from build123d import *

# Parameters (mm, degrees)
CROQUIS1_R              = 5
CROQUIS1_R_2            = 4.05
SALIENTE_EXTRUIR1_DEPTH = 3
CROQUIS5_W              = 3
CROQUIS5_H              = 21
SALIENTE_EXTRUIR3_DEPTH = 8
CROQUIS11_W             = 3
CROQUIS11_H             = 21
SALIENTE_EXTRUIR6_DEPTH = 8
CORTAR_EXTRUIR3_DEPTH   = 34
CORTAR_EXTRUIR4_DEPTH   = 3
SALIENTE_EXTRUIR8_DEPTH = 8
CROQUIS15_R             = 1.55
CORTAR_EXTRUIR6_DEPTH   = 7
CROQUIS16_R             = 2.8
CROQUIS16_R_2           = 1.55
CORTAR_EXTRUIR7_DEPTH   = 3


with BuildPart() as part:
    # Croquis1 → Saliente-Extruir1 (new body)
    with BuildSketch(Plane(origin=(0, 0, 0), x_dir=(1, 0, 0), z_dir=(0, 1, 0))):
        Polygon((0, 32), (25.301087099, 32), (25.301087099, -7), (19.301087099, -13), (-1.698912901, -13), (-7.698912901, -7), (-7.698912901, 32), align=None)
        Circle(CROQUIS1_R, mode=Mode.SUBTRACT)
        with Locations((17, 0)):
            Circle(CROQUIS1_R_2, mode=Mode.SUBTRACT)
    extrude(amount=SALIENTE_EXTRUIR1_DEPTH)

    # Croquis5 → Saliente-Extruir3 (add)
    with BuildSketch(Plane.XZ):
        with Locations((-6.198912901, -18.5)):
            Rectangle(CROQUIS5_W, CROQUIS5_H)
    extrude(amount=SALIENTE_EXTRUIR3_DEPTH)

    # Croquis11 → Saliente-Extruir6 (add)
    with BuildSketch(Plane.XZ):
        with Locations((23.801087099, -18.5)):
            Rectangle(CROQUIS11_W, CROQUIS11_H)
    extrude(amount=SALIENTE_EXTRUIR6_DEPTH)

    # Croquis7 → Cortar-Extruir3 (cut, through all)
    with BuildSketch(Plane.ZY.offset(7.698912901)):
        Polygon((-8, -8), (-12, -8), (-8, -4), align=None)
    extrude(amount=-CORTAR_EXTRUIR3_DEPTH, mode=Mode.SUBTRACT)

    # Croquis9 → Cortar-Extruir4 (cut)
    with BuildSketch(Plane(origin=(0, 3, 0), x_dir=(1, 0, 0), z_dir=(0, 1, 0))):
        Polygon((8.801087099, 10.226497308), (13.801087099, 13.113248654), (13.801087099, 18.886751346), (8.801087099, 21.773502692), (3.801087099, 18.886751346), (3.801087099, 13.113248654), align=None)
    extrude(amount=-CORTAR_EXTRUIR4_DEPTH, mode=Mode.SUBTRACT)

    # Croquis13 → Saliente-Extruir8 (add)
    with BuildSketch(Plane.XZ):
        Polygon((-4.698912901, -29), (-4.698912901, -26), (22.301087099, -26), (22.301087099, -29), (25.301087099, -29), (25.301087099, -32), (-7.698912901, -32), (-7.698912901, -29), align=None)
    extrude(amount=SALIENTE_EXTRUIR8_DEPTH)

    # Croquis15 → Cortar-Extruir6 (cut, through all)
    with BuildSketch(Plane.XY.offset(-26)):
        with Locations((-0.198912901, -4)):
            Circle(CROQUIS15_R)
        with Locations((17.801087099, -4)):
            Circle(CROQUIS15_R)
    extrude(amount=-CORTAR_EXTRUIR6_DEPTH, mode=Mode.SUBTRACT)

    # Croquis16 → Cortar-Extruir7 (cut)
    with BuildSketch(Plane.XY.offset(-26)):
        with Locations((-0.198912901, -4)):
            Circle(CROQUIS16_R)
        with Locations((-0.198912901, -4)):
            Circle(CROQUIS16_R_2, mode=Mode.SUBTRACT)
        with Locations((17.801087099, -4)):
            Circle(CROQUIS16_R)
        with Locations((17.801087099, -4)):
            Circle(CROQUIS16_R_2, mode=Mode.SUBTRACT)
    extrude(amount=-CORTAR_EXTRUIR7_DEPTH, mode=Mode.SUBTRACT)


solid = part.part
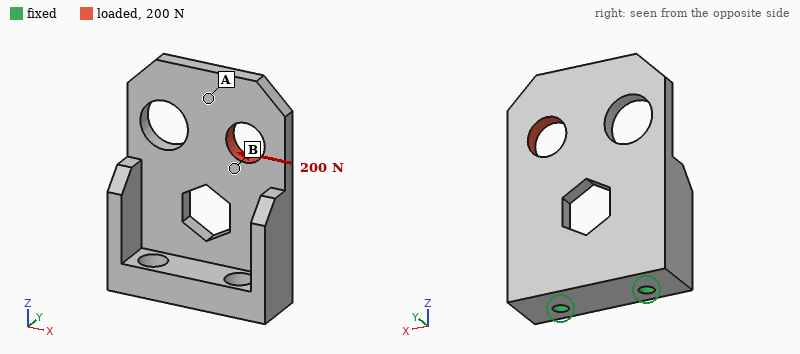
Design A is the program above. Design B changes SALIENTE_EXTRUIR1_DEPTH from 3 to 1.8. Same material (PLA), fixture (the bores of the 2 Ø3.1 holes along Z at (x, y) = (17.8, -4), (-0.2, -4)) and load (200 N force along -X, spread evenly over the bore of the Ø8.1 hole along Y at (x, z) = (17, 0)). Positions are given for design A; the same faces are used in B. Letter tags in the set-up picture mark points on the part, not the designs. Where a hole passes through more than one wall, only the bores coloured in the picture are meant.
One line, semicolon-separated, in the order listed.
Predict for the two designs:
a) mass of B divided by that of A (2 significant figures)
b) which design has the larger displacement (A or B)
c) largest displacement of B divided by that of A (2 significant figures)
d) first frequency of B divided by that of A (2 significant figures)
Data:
0.75; B; 1.3; 0.85
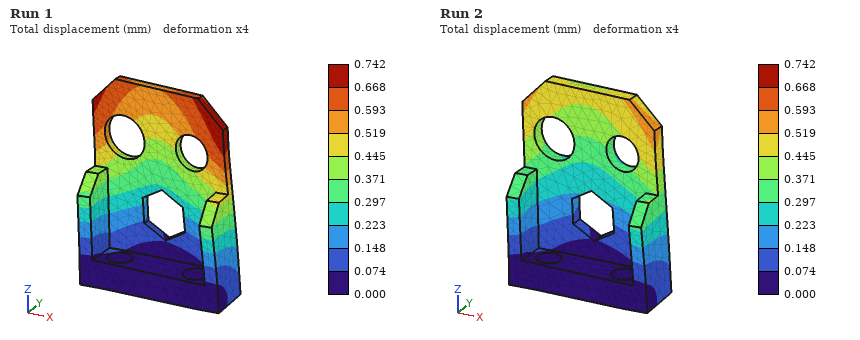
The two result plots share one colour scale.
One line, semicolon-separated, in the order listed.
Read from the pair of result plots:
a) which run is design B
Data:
Run 1
